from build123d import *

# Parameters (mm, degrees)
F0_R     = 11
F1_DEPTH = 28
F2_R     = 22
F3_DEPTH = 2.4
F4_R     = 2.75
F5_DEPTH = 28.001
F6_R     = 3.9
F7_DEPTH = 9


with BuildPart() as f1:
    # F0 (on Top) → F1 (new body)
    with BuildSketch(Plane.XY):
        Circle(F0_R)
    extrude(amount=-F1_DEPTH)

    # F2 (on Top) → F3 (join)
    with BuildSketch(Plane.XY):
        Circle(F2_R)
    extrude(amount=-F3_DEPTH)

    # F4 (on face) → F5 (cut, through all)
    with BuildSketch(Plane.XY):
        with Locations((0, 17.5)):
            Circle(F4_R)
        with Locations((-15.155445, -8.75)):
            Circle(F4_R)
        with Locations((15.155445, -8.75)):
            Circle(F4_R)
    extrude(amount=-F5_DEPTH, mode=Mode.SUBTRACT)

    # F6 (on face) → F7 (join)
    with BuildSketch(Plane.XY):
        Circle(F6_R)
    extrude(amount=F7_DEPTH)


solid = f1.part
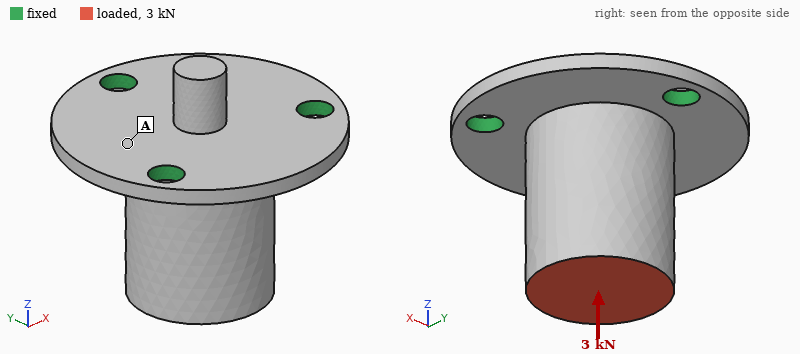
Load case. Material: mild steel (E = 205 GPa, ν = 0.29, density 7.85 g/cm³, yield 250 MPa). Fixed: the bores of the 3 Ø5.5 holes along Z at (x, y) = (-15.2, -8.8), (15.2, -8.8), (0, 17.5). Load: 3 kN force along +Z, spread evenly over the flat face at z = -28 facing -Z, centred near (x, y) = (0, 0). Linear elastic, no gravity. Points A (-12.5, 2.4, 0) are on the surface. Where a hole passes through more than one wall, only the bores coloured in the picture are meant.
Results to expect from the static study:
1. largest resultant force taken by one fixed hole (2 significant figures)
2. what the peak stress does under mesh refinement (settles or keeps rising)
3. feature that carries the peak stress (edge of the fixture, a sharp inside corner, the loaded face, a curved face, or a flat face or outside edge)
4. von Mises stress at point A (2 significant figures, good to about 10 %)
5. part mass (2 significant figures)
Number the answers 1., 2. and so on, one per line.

1. 1.1 kN
2. keeps rising
3. edge of the fixture
4. 40 MPa
5. 110 g
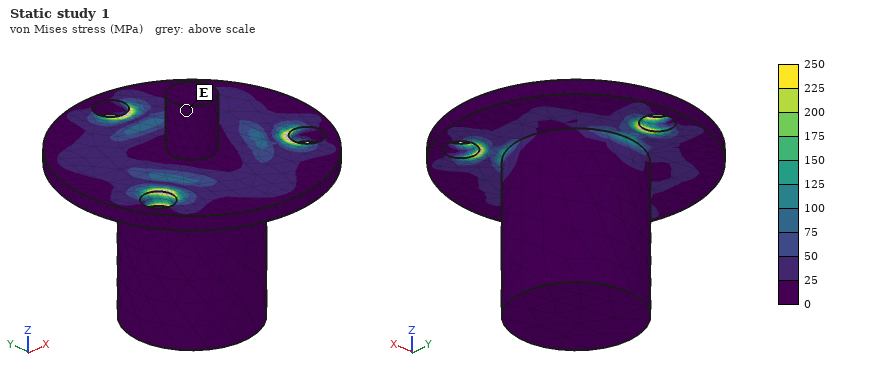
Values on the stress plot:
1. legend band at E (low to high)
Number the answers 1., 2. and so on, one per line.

1. 0 to 25 MPa
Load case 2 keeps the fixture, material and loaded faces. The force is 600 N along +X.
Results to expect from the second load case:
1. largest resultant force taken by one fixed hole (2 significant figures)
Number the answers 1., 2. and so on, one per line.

1. 700 N
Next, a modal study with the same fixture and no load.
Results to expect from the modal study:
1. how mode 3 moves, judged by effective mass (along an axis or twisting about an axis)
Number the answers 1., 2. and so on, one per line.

1. along Z
